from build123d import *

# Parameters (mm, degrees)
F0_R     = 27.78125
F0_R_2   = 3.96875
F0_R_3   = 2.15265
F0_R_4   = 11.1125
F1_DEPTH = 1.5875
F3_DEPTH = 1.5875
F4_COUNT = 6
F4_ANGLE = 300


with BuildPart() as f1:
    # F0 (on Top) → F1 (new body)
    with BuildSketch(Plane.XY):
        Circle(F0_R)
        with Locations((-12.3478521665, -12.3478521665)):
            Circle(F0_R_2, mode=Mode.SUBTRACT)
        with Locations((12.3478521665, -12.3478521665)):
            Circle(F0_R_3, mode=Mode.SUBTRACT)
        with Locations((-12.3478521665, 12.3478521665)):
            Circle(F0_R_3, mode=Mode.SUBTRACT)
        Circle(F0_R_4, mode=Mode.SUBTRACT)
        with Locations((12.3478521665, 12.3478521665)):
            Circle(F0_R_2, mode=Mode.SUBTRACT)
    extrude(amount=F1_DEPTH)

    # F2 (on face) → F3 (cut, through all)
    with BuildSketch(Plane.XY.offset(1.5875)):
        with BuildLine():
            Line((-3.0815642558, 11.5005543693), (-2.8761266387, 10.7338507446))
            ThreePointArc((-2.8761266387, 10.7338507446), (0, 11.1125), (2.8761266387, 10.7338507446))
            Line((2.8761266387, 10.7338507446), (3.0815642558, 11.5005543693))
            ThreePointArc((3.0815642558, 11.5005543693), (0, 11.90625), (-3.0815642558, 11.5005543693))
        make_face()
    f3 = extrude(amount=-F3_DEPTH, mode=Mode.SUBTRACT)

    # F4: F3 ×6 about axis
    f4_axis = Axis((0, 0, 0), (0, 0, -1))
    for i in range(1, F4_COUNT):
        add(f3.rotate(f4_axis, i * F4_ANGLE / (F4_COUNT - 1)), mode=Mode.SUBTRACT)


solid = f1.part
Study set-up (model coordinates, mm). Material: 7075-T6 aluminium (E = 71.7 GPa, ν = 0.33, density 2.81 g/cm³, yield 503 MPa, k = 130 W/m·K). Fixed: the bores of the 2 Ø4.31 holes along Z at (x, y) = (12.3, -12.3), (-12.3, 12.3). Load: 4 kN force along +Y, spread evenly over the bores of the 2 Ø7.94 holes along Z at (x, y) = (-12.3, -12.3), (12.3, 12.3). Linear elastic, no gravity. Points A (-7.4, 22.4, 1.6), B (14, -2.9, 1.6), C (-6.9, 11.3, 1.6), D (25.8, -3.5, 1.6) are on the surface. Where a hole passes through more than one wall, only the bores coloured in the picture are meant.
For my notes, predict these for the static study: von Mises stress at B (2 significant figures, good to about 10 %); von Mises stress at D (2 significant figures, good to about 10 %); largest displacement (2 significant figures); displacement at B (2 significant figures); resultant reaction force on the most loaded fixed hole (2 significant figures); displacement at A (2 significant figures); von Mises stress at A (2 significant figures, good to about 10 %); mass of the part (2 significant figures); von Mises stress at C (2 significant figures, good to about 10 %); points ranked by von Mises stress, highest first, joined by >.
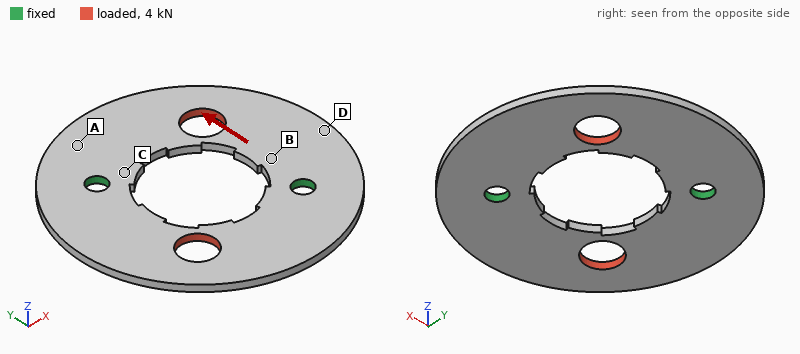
89 MPa
17 MPa
48 µm
16 µm
2.0 kN
13 µm
36 MPa
8.4 g
63 MPa
B > C > A > D
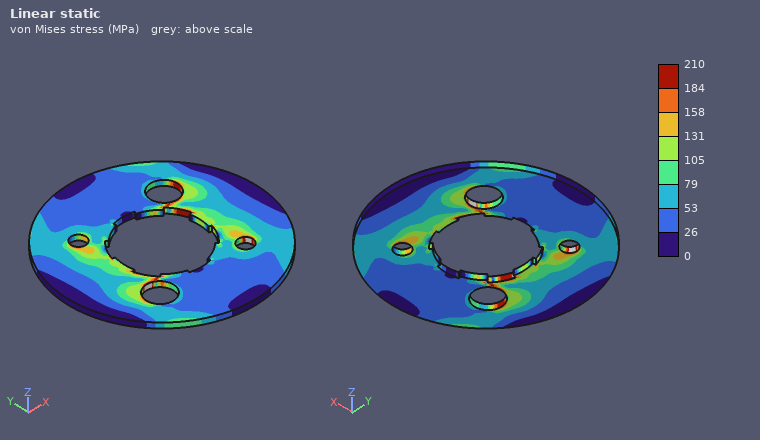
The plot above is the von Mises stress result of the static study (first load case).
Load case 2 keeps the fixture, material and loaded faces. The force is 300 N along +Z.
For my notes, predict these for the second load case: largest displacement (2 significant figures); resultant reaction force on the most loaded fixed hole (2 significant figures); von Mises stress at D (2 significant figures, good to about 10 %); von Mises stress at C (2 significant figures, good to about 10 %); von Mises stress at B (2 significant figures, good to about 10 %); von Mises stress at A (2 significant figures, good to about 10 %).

0.78 mm
150 N
70 MPa
190 MPa
110 MPa
100 MPa
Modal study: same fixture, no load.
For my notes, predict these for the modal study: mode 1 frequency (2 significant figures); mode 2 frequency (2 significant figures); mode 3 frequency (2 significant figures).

1900 Hz
1900 Hz
4300 Hz
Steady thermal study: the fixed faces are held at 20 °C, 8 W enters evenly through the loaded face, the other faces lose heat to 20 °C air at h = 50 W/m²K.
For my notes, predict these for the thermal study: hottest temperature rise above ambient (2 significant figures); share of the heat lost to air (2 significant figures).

15 K
19 %
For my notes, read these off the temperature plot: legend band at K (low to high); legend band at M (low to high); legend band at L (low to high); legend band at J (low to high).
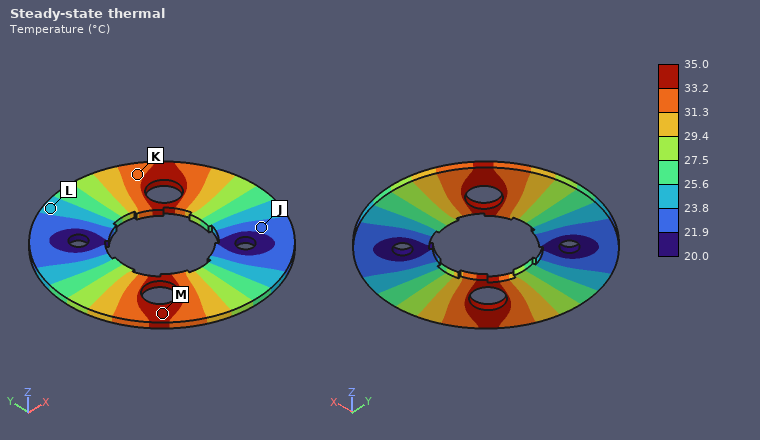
31.3 to 33.2 °C
33.2 to 35.0 °C
23.8 to 25.6 °C
21.9 to 23.8 °C
